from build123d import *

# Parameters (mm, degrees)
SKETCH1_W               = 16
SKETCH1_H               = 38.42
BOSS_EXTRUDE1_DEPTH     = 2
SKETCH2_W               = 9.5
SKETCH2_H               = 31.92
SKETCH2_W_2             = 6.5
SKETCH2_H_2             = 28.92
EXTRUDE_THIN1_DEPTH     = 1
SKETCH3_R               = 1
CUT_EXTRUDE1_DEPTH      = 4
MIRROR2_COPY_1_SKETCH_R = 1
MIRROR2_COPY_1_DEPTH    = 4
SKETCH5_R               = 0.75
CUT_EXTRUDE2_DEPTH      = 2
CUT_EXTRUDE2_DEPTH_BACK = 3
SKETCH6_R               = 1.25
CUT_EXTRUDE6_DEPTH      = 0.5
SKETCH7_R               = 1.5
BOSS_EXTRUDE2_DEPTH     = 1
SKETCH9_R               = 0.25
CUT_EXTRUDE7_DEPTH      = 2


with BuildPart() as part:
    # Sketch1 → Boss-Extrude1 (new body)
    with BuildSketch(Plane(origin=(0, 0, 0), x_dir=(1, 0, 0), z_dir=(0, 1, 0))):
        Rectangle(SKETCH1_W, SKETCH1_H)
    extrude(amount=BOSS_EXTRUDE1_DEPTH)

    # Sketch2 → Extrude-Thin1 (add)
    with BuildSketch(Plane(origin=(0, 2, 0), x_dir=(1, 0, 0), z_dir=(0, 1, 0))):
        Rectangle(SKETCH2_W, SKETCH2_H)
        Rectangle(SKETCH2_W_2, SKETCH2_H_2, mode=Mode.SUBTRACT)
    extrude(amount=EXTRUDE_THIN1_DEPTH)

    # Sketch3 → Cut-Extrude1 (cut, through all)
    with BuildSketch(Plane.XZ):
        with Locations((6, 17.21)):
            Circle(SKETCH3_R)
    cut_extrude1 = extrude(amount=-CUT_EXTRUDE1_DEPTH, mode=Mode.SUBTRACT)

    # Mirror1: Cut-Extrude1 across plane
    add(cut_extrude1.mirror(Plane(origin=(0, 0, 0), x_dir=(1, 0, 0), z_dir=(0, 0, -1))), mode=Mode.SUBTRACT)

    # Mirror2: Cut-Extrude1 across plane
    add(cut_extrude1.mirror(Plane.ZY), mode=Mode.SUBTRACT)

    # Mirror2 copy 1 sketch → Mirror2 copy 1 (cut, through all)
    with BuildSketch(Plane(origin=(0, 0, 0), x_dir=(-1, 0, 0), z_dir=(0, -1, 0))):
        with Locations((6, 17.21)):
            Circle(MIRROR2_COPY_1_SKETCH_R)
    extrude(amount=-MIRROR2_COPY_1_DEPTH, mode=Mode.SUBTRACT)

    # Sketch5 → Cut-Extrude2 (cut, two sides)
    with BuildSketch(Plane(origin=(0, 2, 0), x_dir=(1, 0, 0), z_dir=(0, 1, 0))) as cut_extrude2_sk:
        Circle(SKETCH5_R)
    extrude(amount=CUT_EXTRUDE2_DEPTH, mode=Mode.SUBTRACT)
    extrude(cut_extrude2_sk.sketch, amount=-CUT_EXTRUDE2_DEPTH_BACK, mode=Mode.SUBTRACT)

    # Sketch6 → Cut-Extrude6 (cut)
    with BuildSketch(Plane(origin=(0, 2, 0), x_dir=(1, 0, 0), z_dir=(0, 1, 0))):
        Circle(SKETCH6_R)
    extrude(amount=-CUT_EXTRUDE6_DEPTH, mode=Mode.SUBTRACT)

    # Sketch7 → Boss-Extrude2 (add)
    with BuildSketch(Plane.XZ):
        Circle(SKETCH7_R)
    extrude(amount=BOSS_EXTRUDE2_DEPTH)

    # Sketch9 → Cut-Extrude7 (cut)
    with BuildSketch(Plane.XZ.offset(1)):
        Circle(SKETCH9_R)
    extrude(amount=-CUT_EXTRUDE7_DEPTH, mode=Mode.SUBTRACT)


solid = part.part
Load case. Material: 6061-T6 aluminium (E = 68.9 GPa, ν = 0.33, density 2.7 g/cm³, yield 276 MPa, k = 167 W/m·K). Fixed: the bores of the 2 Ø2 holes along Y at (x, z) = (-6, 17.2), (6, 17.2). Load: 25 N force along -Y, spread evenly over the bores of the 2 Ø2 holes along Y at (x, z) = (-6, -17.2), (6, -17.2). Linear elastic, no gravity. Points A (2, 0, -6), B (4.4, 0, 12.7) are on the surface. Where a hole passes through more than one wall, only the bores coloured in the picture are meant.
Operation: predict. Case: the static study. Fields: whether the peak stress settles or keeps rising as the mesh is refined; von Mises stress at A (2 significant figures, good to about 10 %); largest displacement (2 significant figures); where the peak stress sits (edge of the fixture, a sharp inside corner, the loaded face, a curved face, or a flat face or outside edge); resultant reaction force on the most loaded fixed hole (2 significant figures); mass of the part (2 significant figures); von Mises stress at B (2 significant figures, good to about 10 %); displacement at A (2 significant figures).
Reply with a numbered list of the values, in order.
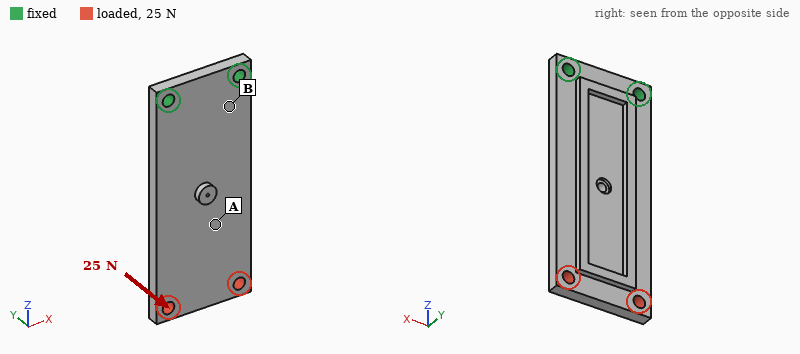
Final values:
1. keeps rising
2. 19 MPa
3. 0.36 mm
4. edge of the fixture
5. 13 N
6. 3.6 g
7. 53 MPa
8. 0.18 mm
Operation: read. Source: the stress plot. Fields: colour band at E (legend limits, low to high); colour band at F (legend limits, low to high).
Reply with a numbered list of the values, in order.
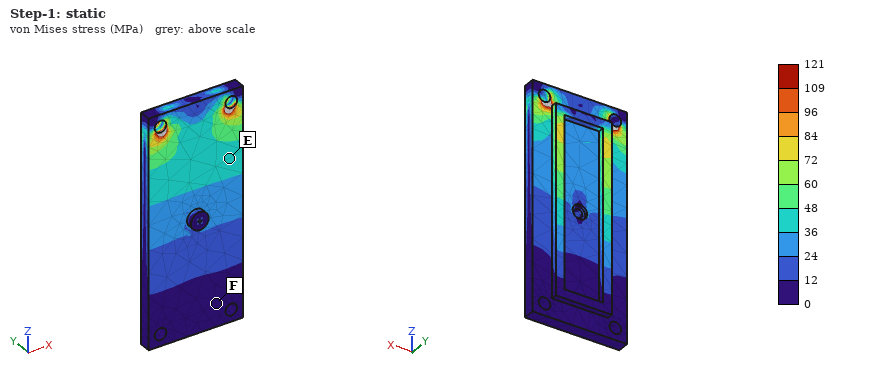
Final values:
1. 36 to 48 MPa
2. 0 to 12 MPa
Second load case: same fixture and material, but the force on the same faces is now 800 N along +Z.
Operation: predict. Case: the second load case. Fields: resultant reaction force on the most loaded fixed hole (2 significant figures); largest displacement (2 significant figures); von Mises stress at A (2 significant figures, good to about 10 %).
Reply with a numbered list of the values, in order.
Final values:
1. 410 N
2. 51 µm
3. 27 MPa
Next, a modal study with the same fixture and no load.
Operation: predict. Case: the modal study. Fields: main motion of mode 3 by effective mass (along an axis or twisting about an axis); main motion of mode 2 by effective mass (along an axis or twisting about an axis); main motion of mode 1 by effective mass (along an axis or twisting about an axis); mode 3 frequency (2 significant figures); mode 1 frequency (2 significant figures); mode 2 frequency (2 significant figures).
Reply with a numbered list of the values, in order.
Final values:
1. along X
2. twisting about Z
3. along Y
4. 8700 Hz
5. 1400 Hz
6. 6200 Hz
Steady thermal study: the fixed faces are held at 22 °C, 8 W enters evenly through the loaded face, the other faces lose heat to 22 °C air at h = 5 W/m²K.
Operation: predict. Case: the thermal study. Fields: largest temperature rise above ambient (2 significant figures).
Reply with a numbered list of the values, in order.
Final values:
1. 53 K
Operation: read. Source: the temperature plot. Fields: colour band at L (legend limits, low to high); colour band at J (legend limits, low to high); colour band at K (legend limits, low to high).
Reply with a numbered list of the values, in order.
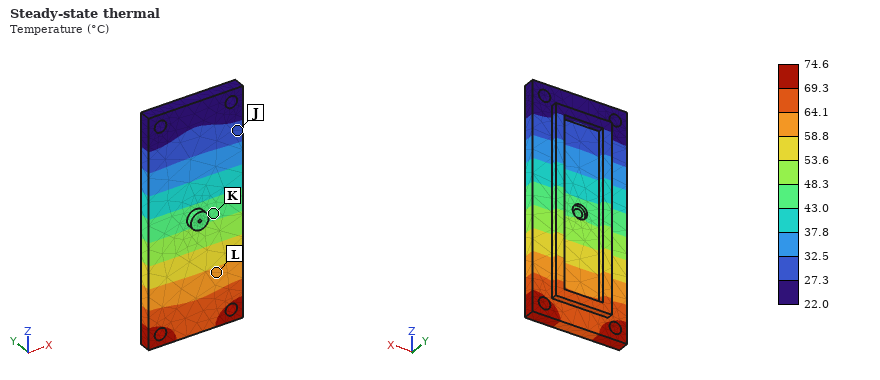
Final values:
1. 58.8 to 64.1 °C
2. 27.3 to 32.5 °C
3. 43.0 to 48.3 °C
